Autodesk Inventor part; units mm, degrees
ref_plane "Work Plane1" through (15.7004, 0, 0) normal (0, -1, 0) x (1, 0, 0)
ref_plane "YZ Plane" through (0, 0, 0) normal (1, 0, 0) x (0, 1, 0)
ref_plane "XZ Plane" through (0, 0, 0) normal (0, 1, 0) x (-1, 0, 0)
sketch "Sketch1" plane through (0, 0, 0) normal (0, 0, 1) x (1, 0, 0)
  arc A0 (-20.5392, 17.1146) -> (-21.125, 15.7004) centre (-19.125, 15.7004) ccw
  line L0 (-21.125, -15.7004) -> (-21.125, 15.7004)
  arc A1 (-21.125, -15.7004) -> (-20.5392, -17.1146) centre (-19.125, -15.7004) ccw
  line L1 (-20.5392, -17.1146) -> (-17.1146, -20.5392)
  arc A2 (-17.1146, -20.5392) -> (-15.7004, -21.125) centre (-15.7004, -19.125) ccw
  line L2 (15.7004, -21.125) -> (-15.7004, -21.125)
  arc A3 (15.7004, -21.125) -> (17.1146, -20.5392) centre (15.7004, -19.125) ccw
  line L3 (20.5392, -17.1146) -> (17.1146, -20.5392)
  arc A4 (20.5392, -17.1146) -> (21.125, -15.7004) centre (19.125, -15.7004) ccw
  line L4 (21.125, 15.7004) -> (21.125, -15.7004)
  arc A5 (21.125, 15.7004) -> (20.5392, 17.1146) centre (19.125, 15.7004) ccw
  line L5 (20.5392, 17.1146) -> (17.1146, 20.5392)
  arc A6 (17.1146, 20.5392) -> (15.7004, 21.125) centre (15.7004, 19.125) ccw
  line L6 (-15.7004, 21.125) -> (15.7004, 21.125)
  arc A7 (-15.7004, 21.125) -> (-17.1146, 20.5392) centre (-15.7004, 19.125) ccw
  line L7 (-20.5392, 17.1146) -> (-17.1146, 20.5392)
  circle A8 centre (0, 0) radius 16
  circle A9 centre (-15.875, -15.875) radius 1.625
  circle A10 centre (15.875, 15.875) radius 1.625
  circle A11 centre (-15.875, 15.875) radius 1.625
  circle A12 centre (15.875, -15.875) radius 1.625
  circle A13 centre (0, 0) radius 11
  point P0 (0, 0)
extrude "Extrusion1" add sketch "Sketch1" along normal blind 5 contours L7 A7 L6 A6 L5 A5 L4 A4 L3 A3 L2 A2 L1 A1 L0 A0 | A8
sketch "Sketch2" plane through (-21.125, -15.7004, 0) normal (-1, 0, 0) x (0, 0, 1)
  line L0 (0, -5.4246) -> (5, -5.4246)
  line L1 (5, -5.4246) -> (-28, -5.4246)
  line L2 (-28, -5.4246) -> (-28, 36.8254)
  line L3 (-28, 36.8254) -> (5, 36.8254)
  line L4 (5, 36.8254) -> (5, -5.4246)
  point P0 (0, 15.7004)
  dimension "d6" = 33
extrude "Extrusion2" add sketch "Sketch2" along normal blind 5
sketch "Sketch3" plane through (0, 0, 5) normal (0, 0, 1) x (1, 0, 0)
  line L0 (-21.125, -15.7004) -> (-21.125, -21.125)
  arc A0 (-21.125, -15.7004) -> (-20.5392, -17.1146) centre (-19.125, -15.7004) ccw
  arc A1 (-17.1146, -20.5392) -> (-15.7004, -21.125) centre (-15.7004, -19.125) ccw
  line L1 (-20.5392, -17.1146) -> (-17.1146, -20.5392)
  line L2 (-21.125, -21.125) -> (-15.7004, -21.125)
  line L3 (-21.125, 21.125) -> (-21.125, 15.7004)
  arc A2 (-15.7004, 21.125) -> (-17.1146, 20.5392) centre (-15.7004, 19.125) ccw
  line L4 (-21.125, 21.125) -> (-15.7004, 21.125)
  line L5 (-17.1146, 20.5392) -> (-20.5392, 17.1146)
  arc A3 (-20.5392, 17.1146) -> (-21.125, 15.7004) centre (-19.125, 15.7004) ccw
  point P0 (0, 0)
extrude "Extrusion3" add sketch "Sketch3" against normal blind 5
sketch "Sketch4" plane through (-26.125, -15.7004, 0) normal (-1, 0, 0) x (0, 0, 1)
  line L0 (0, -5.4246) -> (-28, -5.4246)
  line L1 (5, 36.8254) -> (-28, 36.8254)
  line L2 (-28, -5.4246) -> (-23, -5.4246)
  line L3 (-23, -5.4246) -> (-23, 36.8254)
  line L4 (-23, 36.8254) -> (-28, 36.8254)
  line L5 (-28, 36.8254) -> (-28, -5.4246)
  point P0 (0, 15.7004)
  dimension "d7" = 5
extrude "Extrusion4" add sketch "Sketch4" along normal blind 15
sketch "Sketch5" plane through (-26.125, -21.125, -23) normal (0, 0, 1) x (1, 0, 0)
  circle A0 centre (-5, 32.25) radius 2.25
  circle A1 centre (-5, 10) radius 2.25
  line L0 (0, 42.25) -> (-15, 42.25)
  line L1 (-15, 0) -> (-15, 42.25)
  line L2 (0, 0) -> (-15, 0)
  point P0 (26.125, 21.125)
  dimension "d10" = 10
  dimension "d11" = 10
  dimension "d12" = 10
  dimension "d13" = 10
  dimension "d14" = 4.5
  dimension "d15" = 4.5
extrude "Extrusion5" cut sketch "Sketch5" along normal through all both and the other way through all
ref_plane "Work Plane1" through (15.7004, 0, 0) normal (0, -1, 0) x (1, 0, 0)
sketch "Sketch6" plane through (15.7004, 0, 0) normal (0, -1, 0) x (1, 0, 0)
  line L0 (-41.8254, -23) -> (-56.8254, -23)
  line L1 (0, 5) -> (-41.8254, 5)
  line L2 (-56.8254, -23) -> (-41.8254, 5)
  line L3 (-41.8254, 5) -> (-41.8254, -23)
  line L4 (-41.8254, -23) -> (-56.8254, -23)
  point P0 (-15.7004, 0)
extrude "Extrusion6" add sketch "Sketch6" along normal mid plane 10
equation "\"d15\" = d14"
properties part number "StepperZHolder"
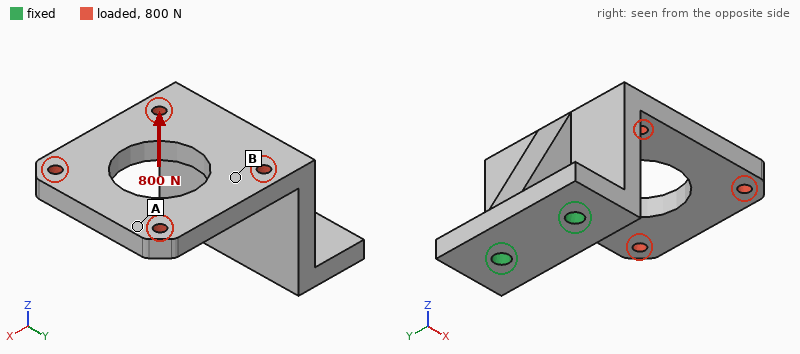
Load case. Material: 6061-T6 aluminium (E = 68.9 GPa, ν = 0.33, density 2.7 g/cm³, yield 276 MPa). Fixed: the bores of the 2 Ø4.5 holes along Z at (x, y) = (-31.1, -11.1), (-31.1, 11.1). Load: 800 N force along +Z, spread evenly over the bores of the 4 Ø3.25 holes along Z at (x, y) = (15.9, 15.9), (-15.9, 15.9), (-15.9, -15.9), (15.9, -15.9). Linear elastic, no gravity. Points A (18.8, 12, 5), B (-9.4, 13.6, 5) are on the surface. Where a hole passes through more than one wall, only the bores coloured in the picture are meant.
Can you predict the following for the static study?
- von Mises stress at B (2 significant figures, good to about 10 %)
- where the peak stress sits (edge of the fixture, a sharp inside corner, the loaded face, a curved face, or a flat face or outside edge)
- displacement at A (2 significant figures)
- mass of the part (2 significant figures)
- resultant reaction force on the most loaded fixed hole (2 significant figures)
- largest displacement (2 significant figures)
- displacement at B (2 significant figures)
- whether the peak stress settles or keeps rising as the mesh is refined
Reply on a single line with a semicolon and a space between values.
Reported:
91 MPa; edge of the fixture; 0.74 mm; 51 g; 400 N; 0.80 mm; 0.22 mm; keeps rising
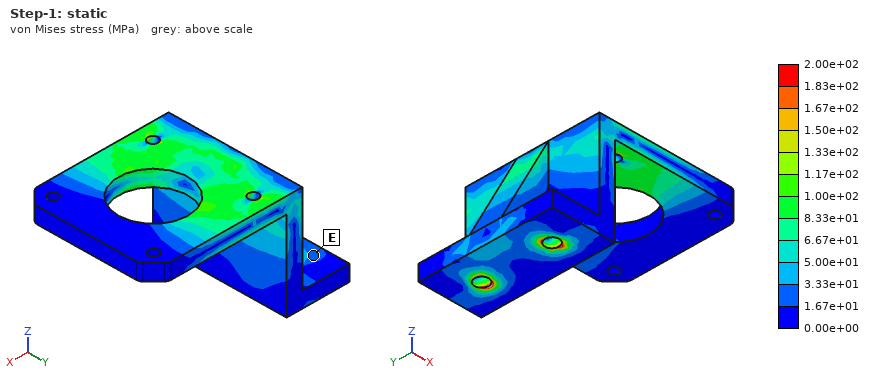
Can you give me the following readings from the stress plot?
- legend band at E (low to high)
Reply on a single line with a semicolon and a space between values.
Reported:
1.67e+01 to 3.33e+01 MPa
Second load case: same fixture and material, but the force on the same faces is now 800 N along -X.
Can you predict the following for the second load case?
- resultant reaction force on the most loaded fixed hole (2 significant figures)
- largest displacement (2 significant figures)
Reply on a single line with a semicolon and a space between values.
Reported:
410 N; 0.21 mm
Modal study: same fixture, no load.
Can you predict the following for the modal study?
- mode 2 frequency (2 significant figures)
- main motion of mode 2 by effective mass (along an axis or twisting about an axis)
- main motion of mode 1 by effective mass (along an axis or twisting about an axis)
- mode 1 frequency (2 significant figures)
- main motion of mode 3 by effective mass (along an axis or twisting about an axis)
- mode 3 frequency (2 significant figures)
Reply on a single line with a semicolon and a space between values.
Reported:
2400 Hz; along Y; along Z; 1400 Hz; along X; 3500 Hz
